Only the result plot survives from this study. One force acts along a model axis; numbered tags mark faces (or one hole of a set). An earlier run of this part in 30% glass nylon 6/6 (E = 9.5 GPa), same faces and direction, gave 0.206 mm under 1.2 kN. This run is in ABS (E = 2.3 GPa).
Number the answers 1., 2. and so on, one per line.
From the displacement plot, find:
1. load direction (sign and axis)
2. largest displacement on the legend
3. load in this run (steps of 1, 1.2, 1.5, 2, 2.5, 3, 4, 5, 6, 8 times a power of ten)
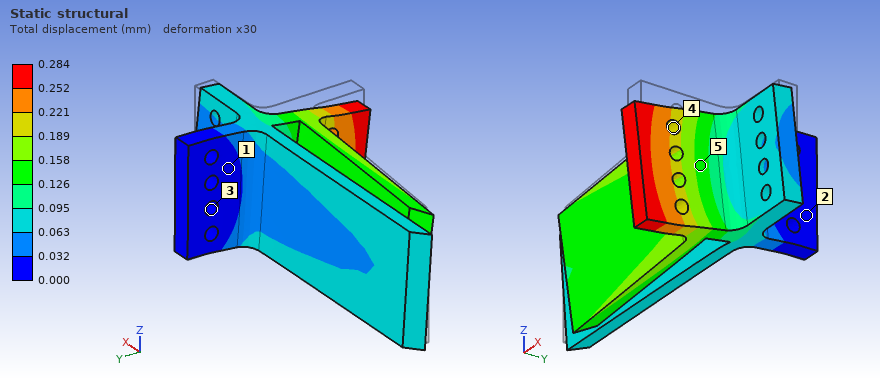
1. -Z
2. 0.284 mm
3. 400 N
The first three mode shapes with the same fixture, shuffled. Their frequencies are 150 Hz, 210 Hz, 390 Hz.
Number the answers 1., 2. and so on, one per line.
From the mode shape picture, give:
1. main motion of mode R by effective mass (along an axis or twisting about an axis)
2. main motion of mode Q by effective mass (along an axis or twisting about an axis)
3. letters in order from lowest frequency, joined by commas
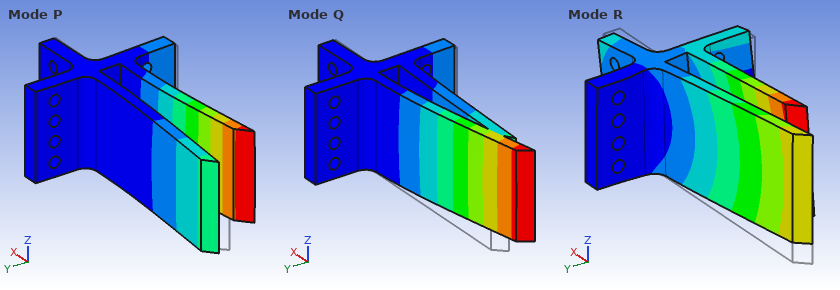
1. along Z
2. along Y
3. Q, P, R
